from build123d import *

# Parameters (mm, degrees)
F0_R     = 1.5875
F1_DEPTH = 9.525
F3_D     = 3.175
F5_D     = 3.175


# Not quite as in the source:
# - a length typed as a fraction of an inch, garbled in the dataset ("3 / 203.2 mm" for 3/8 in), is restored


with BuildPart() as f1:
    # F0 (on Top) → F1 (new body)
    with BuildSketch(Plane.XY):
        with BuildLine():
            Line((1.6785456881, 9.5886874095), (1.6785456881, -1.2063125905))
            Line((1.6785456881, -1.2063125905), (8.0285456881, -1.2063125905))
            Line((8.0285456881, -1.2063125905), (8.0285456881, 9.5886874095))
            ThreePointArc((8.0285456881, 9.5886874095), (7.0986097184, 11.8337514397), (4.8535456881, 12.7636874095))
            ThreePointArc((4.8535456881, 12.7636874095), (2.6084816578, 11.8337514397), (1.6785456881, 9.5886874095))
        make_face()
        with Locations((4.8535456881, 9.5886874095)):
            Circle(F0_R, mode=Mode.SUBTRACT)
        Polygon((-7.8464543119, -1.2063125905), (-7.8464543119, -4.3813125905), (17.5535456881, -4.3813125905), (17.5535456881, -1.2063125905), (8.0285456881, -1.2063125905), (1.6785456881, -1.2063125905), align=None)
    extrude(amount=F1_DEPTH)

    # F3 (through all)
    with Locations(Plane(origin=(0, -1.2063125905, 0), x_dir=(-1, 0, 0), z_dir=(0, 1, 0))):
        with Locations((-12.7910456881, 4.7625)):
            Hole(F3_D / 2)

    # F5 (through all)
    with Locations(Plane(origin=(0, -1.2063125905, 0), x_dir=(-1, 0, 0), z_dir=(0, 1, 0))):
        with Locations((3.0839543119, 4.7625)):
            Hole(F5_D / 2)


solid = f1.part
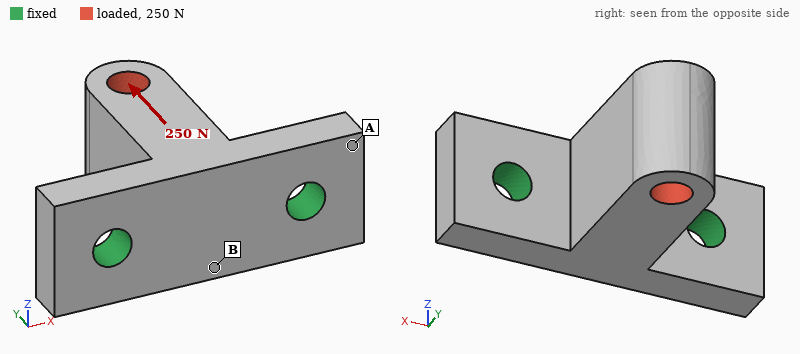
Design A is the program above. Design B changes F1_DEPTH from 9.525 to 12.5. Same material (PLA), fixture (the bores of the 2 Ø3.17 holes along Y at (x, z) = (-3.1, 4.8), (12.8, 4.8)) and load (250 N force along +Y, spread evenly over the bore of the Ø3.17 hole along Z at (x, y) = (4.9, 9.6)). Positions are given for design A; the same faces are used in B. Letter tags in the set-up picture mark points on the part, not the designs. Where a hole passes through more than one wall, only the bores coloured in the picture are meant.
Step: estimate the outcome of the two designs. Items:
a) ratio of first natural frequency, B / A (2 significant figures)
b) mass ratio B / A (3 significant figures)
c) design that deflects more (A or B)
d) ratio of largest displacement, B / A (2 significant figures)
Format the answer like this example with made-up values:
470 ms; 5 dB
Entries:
0.96; 1.32; B; 1.7
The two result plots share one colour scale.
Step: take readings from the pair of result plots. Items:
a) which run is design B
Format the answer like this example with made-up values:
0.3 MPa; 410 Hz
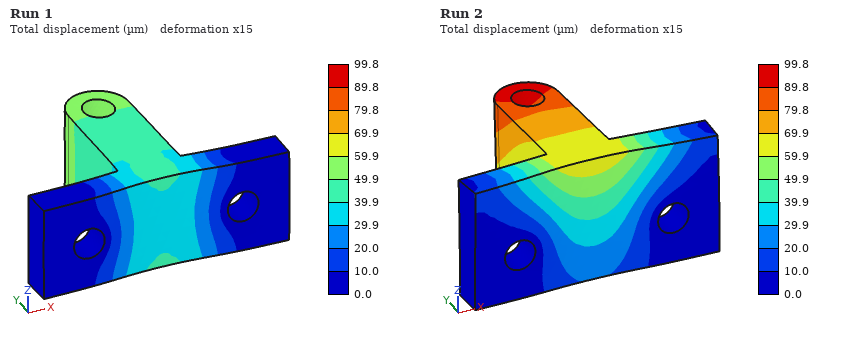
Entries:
Run 2
